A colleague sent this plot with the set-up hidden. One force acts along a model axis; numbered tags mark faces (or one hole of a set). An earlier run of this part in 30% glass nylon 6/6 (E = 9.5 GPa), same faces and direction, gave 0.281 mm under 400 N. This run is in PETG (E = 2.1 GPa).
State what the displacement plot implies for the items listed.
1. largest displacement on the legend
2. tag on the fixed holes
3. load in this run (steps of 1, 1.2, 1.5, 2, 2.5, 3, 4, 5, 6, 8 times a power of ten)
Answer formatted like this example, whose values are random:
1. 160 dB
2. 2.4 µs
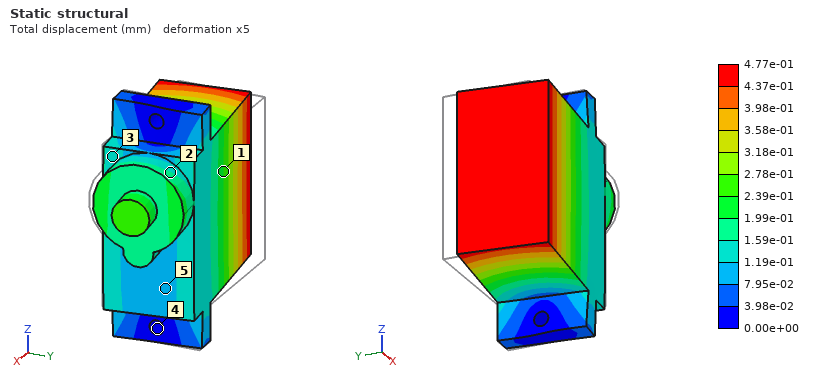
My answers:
1. 4.77e-01 mm
2. 4
3. 150 N
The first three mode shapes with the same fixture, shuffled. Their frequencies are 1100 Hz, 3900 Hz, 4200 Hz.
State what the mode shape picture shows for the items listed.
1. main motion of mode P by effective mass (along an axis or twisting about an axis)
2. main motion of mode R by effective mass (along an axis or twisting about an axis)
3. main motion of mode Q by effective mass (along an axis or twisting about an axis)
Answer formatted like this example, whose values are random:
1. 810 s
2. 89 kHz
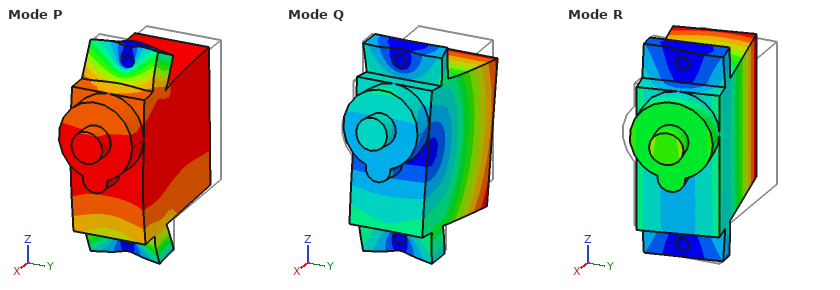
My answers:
1. along X
2. along Y
3. along Z
